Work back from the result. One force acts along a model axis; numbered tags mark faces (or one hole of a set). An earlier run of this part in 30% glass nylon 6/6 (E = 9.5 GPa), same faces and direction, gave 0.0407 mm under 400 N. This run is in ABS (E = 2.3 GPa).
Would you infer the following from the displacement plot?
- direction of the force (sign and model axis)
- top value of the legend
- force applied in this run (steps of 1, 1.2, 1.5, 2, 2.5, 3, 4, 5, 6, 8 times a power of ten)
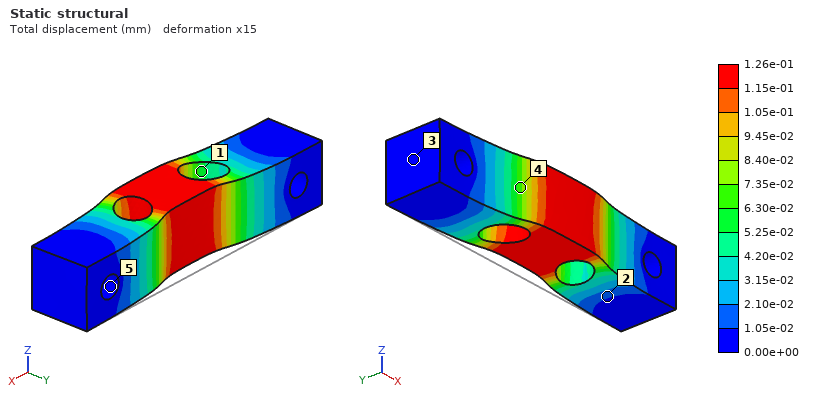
-Y
1.26e-01 mm
300 N
